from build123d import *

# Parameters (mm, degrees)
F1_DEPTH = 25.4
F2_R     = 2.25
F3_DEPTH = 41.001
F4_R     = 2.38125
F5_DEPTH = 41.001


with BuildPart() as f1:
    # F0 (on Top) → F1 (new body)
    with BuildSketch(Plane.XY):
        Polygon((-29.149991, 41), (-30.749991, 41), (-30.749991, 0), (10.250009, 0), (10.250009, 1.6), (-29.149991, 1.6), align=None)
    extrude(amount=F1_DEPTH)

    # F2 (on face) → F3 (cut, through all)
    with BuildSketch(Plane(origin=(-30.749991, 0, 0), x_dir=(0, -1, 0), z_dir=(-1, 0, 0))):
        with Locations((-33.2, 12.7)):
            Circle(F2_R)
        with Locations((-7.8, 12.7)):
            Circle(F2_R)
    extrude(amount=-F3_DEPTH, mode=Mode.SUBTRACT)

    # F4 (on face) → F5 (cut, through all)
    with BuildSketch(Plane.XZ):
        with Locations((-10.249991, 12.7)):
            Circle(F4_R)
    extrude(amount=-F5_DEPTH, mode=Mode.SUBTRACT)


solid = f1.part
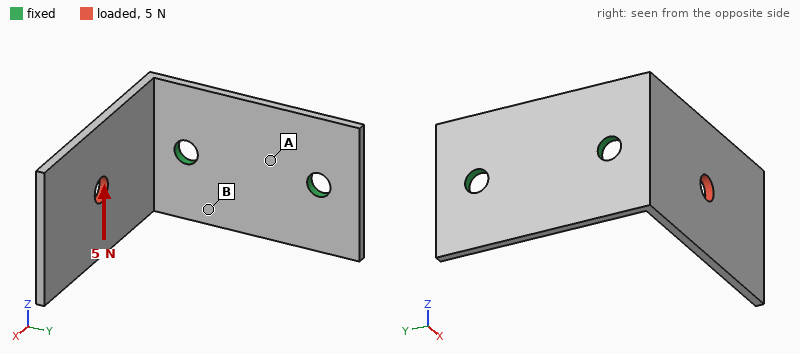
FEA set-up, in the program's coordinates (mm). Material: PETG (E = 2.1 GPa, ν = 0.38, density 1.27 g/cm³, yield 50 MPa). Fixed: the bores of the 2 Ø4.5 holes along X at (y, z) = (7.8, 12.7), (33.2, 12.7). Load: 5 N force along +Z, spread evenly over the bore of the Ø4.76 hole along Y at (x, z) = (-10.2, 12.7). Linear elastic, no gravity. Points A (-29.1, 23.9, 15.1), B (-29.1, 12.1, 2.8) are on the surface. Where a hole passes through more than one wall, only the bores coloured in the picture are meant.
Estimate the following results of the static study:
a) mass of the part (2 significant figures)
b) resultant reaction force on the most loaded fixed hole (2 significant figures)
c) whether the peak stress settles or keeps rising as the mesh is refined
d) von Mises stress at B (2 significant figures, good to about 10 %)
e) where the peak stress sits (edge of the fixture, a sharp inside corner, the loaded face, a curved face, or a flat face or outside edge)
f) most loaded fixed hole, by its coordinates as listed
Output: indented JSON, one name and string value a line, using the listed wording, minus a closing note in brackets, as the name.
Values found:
{
  "mass of the part": "4.0 g",
  "resultant reaction force on the most loaded fixed hole": "5.9 N",
  "whether the peak stress settles or keeps rising as the mesh is refined": "keeps rising",
  "von Mises stress at B": "2.3 MPa",
  "where the peak stress sits": "edge of the fixture",
  "most loaded fixed hole, by its coordinates as listed": "(7.8, 12.7)"
}
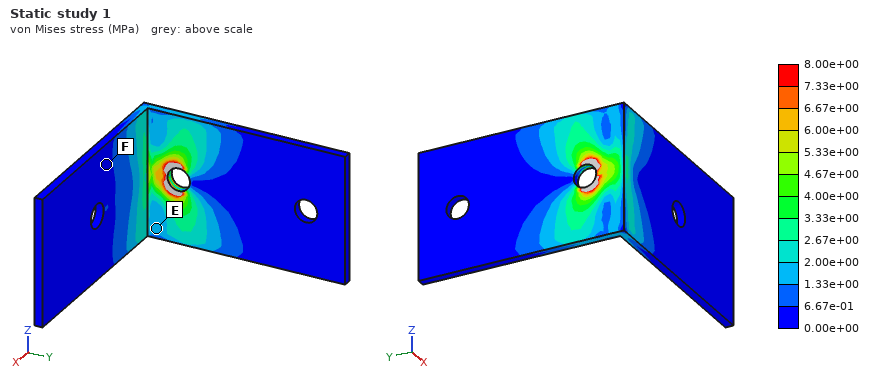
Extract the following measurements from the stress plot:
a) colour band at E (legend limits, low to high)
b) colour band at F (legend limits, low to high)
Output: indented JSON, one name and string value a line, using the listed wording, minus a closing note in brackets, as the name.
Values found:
{
  "colour band at E": "1.33e+00 to 2.00e+00 MPa",
  "colour band at F": "0.00e+00 to 6.67e-01 MPa"
}
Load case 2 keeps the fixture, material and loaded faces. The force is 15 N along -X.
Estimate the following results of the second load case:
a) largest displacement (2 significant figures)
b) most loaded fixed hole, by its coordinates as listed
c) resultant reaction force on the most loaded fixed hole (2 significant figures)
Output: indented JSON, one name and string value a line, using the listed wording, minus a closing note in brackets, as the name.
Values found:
{
  "largest displacement": "0.65 mm",
  "most loaded fixed hole, by its coordinates as listed": "(7.8, 12.7)",
  "resultant reaction force on the most loaded fixed hole": "15 N"
}
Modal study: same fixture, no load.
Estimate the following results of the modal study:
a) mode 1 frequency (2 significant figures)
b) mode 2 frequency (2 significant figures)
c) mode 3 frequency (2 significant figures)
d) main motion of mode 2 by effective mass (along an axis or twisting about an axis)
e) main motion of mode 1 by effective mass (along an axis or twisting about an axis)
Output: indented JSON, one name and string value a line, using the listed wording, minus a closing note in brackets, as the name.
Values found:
{
  "mode 1 frequency": "170 Hz",
  "mode 2 frequency": "360 Hz",
  "mode 3 frequency": "670 Hz",
  "main motion of mode 2 by effective mass": "along Z",
  "main motion of mode 1 by effective mass": "along Y"
}
